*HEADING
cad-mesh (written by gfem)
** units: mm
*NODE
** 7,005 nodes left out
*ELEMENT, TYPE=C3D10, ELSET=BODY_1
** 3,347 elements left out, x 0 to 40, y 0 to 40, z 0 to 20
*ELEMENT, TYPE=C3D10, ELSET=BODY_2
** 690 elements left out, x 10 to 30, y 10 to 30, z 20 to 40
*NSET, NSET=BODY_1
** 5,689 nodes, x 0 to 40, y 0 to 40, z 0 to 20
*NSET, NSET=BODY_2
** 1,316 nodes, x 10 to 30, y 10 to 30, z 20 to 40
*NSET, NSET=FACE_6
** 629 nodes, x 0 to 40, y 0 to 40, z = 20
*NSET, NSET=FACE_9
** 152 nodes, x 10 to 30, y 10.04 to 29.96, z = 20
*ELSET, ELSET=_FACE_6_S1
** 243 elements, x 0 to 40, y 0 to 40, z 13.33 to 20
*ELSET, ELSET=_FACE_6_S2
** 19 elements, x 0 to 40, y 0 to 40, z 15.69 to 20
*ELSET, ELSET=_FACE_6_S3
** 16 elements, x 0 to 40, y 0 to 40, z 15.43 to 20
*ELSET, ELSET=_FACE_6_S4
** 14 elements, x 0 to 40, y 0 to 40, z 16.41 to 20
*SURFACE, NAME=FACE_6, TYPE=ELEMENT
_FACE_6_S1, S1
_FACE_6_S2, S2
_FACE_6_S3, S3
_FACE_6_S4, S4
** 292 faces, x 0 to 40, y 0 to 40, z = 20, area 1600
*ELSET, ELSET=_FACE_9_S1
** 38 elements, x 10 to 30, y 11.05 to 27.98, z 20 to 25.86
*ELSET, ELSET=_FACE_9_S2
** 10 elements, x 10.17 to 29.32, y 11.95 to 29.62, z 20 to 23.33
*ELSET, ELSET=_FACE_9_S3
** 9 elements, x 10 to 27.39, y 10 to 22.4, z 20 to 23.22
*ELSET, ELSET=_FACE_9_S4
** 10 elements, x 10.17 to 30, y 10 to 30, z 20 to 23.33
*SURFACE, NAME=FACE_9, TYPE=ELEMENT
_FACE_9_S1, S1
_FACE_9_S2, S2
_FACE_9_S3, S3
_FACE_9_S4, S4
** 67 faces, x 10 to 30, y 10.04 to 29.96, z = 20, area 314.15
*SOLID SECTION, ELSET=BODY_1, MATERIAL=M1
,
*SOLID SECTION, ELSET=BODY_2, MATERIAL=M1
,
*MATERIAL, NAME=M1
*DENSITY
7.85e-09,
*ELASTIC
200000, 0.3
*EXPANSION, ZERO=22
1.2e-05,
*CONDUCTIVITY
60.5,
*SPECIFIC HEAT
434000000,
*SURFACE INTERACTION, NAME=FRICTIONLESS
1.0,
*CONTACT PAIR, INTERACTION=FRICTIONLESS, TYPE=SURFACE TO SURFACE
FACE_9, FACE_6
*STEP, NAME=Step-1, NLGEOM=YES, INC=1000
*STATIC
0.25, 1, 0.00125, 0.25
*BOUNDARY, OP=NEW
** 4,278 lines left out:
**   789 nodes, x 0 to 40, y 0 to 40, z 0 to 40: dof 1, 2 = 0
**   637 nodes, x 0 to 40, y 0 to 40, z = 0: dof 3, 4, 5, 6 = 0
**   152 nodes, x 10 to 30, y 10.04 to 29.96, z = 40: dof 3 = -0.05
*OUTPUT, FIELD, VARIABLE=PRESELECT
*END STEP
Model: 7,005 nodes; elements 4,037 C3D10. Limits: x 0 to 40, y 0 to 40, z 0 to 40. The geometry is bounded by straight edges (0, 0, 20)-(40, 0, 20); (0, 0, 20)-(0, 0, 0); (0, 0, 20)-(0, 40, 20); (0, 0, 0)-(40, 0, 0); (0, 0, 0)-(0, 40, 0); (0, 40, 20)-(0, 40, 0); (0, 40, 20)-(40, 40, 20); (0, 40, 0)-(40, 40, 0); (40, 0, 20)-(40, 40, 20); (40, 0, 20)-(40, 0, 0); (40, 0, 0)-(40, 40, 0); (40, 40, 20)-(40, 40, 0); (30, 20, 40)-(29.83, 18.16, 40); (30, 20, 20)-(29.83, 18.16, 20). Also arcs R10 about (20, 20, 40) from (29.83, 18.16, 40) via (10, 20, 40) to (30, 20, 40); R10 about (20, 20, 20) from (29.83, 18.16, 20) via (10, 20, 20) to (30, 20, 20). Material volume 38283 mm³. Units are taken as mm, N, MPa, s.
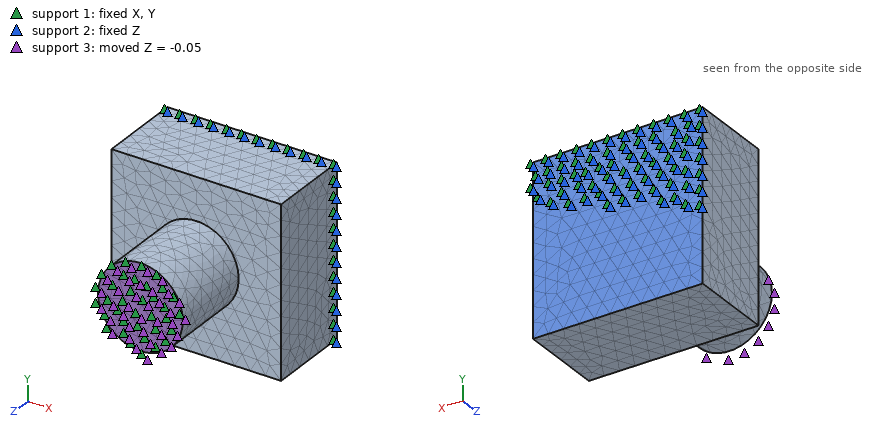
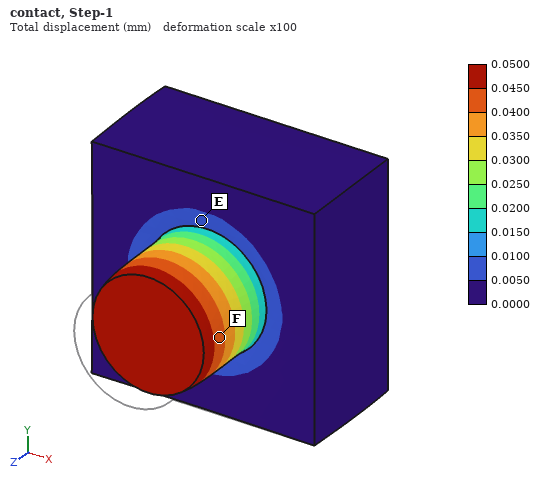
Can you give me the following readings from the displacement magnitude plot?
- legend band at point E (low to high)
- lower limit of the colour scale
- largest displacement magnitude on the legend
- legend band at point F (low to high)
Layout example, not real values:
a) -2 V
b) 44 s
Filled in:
a) 0.0050 to 0.0100 mm
b) 0.0000 mm
c) 0.0500 mm
d) 0.0400 to 0.0450 mm
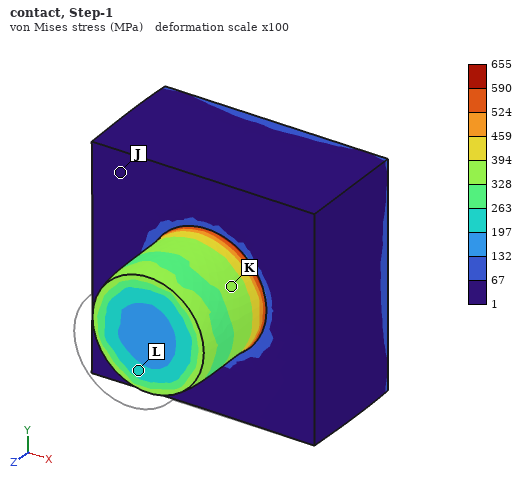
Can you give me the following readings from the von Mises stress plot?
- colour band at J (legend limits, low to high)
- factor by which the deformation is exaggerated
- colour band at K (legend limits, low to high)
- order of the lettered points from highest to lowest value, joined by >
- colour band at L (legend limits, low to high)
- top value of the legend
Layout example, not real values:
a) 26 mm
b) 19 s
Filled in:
a) 1 to 67 MPa
b) 100
c) 328 to 394 MPa
d) K > L > J
e) 197 to 263 MPa
f) 655 MPa
